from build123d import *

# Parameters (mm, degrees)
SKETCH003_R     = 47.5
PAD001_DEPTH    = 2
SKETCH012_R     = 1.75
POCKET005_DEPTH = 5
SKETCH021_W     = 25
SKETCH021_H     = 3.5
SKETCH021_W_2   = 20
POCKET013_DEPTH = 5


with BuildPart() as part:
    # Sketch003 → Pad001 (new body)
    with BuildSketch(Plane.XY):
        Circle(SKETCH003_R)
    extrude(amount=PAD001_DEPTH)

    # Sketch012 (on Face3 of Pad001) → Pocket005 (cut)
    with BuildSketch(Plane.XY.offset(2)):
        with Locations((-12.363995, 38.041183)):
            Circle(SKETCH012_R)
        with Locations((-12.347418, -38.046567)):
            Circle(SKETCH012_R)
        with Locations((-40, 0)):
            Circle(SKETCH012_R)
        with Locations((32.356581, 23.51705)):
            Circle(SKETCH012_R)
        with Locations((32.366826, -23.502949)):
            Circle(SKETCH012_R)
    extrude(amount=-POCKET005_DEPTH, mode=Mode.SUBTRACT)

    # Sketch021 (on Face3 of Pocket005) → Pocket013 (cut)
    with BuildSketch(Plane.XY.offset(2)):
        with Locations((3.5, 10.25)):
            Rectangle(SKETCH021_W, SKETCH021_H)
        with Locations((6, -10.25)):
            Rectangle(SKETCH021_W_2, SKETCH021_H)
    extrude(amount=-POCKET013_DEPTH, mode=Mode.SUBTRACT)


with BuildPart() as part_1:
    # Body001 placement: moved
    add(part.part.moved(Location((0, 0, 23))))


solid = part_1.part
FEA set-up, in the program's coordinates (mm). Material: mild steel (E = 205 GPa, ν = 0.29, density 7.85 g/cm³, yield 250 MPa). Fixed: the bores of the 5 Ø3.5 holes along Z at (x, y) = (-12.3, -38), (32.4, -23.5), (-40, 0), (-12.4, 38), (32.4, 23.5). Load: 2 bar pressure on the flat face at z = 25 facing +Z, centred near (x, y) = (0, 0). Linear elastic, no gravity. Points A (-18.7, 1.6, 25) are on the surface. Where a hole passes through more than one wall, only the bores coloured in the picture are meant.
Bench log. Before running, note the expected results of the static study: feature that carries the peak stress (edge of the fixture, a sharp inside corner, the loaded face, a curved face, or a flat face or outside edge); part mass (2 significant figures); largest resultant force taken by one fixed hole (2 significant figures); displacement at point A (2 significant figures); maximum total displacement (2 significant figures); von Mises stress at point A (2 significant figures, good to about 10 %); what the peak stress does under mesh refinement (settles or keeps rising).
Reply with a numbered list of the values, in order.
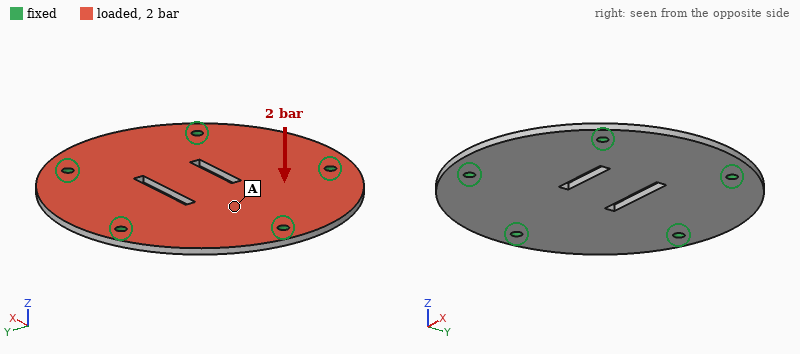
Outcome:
1. edge of the fixture
2. 110 g
3. 280 N
4. 53 µm
5. 84 µm
6. 22 MPa
7. keeps rising
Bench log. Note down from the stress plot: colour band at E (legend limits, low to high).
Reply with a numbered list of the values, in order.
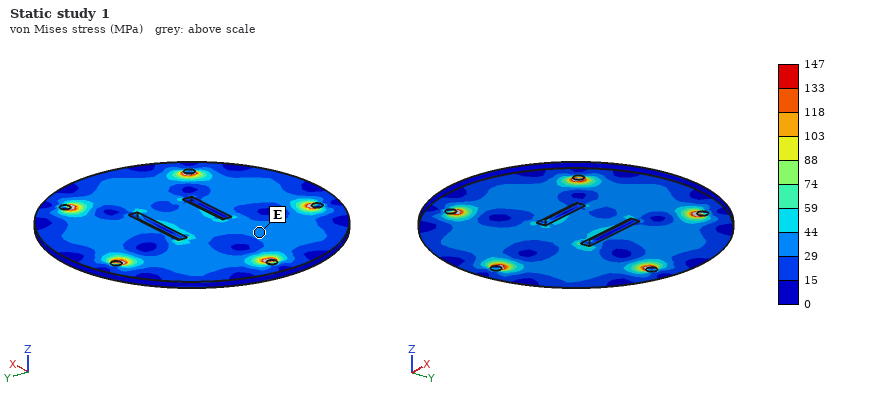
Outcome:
1. 29 to 44 MPa
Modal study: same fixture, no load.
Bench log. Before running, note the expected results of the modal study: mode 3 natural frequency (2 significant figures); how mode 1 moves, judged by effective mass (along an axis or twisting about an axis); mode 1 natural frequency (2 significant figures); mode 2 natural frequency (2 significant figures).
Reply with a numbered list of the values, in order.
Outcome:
1. 4000 Hz
2. along Z
3. 2400 Hz
4. 4000 Hz
